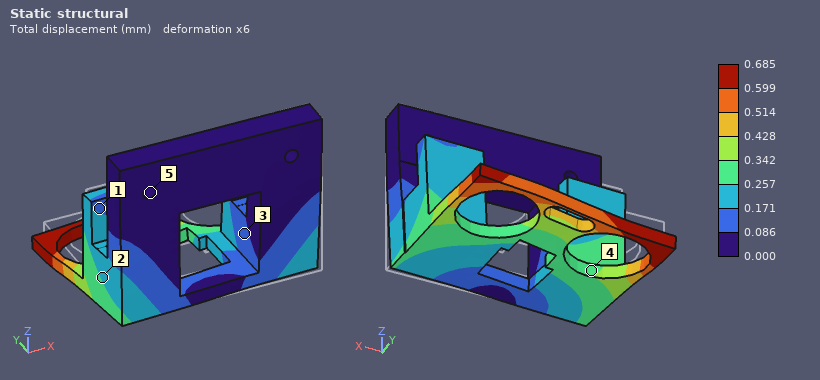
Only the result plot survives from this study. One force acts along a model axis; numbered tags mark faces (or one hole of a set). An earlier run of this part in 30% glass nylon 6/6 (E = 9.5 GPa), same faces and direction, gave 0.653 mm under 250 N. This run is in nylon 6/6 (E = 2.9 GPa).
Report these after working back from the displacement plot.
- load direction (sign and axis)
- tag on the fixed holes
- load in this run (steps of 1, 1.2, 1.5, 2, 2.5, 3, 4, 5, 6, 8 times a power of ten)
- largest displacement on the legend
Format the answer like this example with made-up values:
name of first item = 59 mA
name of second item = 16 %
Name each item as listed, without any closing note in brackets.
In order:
load direction = -X
tag on the fixed holes = 5
load in this run = 80 N
largest displacement on the legend = 0.685 mm
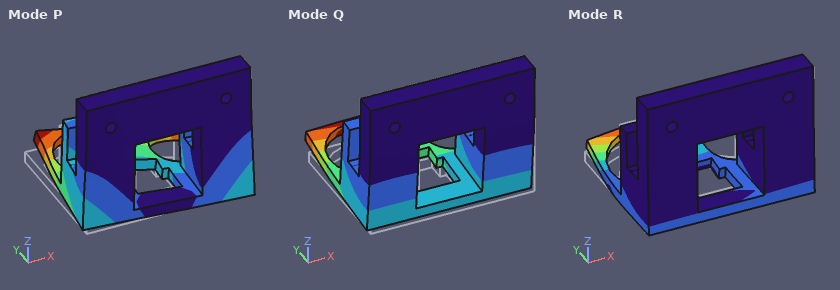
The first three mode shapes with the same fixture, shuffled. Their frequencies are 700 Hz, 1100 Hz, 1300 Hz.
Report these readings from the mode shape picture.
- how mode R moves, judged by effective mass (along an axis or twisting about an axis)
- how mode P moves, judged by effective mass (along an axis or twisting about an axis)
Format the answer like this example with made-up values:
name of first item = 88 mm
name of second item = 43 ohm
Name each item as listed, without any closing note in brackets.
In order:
how mode R moves, judged by effective mass = along Y
how mode P moves, judged by effective mass = along X
